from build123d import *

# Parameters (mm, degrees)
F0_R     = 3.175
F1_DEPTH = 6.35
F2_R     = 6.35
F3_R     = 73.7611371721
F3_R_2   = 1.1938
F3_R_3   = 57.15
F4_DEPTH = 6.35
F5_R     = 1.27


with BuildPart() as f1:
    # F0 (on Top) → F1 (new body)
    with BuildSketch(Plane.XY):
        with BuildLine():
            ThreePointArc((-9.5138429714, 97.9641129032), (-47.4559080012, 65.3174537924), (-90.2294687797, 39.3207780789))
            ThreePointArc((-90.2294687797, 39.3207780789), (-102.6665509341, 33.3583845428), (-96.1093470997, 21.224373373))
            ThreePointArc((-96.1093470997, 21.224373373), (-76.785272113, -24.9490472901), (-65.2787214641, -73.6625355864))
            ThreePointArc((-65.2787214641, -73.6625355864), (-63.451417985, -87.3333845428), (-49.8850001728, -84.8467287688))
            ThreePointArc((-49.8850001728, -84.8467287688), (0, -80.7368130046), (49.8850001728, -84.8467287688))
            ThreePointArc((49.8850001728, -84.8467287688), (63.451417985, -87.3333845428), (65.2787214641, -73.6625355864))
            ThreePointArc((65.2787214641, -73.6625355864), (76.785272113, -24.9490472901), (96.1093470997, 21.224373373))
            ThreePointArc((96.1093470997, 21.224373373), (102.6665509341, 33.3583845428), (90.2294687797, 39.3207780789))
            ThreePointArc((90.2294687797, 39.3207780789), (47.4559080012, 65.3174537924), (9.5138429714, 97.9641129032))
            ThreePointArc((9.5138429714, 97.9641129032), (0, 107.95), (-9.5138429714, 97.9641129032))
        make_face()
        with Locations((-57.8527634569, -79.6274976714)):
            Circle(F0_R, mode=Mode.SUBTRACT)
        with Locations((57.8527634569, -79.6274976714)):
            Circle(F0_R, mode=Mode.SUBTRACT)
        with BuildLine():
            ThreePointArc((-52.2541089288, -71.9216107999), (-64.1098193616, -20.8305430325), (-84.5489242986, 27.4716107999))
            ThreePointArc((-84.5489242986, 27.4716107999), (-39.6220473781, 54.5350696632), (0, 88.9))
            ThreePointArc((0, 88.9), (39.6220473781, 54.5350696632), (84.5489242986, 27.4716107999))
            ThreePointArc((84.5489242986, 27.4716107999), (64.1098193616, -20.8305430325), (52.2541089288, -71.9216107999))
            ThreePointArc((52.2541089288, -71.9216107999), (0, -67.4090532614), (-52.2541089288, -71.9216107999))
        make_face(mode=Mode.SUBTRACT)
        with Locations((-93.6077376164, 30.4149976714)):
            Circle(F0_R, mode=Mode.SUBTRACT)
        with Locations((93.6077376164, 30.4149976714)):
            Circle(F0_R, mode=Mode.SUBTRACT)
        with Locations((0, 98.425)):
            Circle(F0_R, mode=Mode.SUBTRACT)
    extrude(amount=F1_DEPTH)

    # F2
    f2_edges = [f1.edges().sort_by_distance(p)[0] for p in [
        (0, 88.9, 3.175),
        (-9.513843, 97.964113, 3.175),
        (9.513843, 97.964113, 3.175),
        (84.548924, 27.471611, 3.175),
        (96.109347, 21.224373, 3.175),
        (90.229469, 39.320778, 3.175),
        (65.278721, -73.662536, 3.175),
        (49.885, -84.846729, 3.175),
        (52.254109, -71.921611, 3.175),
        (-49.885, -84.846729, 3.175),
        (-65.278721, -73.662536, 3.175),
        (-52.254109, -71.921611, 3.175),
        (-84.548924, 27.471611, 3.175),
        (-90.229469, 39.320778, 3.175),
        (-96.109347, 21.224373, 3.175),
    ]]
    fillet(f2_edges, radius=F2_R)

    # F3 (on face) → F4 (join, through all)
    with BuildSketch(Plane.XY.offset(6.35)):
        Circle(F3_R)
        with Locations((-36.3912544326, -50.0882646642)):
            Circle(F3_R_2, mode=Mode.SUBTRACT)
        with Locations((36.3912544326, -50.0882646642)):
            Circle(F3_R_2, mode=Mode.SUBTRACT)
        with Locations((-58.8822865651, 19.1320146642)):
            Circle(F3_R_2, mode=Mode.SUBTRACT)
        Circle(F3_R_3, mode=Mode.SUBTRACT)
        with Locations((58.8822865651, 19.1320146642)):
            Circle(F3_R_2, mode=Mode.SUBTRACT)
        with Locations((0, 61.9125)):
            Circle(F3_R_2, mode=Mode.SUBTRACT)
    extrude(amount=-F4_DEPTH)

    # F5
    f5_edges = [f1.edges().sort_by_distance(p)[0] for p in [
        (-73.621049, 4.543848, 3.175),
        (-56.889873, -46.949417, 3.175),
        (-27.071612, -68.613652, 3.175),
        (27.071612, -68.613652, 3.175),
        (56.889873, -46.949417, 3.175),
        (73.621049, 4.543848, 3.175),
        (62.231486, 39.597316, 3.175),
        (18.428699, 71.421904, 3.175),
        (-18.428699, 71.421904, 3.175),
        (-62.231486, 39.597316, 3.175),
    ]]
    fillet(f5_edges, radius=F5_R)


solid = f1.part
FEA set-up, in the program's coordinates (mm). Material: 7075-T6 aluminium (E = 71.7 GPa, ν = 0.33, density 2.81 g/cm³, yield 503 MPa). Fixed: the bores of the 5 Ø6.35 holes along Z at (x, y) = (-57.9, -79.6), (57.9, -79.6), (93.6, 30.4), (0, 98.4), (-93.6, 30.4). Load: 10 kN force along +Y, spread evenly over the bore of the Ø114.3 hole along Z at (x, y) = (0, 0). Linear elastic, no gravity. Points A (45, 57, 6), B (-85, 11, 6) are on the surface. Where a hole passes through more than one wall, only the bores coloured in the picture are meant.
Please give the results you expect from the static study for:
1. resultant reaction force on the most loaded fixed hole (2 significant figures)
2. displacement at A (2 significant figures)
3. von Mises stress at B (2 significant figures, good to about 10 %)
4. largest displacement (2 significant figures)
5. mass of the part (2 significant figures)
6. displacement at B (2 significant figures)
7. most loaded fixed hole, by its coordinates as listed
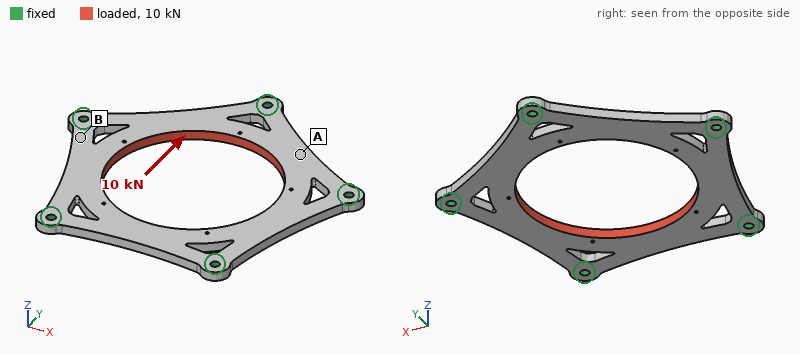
2.7 kN
20 µm
14 MPa
23 µm
240 g
6.3 µm
(0, 98.4)
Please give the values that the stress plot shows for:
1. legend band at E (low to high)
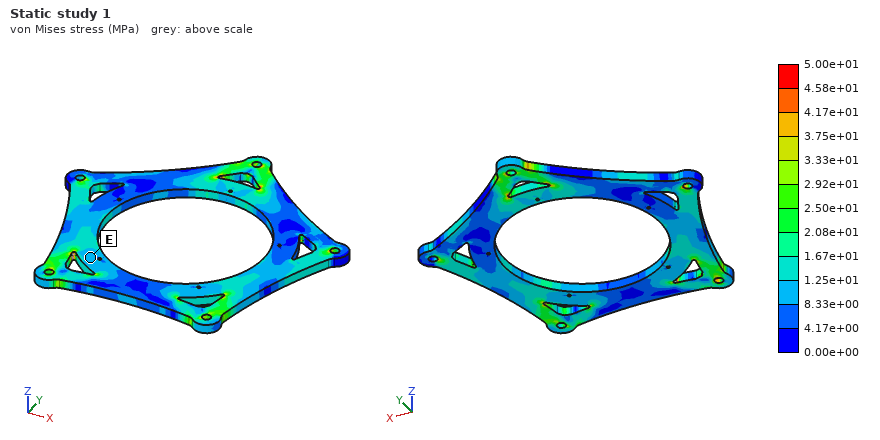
8.33e+00 to 1.25e+01 MPa
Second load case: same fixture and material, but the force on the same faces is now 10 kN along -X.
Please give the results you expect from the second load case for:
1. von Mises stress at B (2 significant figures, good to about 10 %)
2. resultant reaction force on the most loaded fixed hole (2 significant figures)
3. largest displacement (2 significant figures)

18 MPa
2.6 kN
23 µm
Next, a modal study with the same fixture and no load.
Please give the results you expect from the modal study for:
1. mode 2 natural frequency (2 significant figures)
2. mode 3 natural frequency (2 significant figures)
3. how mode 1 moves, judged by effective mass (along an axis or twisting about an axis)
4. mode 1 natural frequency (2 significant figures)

2100 Hz
2100 Hz
along Z
1700 Hz
